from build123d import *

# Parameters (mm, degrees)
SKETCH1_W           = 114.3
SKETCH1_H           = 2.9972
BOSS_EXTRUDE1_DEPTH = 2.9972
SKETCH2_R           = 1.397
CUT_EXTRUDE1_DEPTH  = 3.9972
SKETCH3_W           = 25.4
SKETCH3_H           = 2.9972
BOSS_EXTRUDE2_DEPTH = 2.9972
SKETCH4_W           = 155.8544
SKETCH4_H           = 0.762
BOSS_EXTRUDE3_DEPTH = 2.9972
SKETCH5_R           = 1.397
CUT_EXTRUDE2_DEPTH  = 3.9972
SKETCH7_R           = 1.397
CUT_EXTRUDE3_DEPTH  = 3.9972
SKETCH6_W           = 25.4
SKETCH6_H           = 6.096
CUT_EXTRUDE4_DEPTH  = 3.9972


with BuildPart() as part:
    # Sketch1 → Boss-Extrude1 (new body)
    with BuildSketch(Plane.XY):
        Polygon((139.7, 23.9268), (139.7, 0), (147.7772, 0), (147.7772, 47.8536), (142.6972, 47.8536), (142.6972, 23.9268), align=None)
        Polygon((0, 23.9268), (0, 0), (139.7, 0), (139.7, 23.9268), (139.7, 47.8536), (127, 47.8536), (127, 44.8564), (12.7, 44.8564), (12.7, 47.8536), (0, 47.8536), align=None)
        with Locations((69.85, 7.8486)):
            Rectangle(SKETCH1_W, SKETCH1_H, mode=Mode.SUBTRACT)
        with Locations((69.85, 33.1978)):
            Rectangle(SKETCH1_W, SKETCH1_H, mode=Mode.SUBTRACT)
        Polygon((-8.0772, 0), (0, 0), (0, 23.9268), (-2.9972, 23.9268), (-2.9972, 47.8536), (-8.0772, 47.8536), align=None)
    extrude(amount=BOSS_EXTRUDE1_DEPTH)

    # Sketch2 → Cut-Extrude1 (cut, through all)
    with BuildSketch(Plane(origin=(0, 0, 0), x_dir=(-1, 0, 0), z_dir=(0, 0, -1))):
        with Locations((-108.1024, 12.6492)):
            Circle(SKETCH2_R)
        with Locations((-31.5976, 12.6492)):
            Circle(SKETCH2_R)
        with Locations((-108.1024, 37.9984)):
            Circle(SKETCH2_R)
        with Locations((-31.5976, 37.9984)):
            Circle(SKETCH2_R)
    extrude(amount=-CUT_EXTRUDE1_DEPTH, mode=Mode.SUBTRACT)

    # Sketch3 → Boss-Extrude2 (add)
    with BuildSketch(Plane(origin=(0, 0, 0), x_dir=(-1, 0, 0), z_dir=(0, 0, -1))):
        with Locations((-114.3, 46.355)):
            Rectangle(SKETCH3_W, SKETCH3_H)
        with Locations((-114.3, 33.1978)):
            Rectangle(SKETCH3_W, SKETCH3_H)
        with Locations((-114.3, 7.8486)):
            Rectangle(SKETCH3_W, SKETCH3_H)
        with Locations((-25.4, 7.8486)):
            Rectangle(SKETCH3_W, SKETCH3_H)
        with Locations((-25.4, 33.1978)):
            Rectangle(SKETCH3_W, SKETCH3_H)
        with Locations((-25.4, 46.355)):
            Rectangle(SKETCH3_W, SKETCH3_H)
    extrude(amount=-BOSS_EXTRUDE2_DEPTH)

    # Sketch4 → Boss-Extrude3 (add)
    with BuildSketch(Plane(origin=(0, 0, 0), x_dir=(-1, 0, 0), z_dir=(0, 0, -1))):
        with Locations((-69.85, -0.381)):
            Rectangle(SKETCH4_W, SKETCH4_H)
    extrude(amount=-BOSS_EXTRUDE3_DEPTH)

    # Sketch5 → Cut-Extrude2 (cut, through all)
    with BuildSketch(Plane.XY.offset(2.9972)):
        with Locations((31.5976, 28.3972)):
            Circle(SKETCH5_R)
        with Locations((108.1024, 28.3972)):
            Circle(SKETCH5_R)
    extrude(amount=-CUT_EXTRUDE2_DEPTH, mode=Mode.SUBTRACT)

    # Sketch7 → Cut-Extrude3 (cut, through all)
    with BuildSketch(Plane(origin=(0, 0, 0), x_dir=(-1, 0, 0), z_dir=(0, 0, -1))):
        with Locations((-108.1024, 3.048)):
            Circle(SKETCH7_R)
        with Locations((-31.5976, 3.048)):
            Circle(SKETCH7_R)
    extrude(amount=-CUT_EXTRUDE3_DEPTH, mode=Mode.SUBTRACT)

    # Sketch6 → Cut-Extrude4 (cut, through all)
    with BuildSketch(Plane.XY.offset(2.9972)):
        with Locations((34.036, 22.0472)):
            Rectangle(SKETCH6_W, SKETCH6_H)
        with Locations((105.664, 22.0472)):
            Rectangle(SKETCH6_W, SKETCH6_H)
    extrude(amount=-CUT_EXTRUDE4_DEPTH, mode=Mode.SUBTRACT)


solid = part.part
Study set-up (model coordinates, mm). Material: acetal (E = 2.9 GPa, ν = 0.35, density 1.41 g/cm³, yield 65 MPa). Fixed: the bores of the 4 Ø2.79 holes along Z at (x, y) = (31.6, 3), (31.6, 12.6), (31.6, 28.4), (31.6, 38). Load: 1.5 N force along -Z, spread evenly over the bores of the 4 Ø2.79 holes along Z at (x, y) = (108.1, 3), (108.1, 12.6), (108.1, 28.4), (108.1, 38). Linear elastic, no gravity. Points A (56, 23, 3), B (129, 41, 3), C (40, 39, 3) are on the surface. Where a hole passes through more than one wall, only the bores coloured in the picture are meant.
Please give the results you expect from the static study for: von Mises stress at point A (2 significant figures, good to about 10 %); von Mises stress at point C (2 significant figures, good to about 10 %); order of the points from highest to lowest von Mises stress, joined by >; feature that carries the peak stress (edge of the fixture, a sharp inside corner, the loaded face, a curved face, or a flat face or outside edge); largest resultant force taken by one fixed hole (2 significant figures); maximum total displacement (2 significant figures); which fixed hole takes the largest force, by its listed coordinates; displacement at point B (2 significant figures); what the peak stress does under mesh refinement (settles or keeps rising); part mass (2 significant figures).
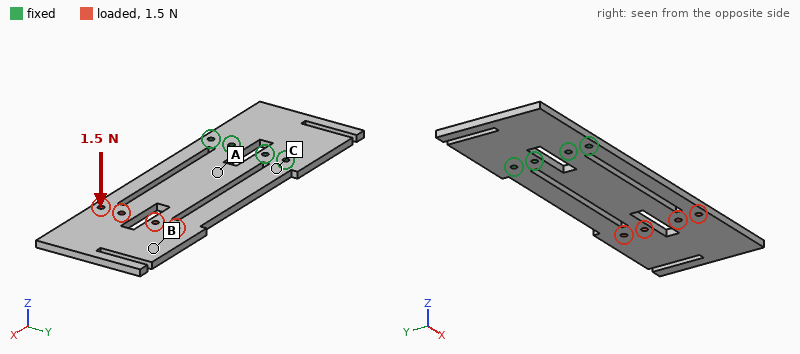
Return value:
1.1 MPa
1.7 MPa
C > A > B
edge of the fixture
0.77 N
1.6 mm
(31.6, 12.6)
1.3 mm
keeps rising
27 g
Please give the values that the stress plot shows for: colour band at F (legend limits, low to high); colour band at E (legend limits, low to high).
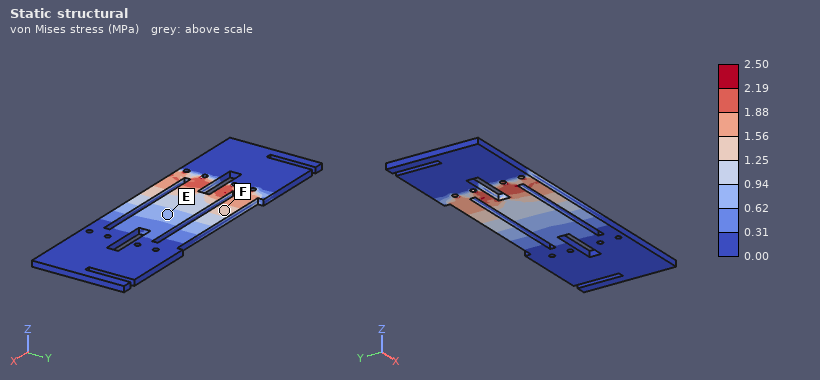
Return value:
1.25 to 1.56 MPa
0.62 to 0.94 MPa
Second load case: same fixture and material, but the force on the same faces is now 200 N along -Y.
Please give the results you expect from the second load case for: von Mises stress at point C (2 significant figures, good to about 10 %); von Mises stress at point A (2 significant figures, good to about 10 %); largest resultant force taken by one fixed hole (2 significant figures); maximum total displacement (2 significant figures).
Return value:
6.2 MPa
7.8 MPa
340 N
1.7 mm
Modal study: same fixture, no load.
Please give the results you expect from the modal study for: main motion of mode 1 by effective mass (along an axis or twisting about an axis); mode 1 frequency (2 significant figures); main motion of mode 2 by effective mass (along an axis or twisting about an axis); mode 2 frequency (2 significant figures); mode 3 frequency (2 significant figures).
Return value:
along Z
48 Hz
twisting about X
230 Hz
310 Hz
